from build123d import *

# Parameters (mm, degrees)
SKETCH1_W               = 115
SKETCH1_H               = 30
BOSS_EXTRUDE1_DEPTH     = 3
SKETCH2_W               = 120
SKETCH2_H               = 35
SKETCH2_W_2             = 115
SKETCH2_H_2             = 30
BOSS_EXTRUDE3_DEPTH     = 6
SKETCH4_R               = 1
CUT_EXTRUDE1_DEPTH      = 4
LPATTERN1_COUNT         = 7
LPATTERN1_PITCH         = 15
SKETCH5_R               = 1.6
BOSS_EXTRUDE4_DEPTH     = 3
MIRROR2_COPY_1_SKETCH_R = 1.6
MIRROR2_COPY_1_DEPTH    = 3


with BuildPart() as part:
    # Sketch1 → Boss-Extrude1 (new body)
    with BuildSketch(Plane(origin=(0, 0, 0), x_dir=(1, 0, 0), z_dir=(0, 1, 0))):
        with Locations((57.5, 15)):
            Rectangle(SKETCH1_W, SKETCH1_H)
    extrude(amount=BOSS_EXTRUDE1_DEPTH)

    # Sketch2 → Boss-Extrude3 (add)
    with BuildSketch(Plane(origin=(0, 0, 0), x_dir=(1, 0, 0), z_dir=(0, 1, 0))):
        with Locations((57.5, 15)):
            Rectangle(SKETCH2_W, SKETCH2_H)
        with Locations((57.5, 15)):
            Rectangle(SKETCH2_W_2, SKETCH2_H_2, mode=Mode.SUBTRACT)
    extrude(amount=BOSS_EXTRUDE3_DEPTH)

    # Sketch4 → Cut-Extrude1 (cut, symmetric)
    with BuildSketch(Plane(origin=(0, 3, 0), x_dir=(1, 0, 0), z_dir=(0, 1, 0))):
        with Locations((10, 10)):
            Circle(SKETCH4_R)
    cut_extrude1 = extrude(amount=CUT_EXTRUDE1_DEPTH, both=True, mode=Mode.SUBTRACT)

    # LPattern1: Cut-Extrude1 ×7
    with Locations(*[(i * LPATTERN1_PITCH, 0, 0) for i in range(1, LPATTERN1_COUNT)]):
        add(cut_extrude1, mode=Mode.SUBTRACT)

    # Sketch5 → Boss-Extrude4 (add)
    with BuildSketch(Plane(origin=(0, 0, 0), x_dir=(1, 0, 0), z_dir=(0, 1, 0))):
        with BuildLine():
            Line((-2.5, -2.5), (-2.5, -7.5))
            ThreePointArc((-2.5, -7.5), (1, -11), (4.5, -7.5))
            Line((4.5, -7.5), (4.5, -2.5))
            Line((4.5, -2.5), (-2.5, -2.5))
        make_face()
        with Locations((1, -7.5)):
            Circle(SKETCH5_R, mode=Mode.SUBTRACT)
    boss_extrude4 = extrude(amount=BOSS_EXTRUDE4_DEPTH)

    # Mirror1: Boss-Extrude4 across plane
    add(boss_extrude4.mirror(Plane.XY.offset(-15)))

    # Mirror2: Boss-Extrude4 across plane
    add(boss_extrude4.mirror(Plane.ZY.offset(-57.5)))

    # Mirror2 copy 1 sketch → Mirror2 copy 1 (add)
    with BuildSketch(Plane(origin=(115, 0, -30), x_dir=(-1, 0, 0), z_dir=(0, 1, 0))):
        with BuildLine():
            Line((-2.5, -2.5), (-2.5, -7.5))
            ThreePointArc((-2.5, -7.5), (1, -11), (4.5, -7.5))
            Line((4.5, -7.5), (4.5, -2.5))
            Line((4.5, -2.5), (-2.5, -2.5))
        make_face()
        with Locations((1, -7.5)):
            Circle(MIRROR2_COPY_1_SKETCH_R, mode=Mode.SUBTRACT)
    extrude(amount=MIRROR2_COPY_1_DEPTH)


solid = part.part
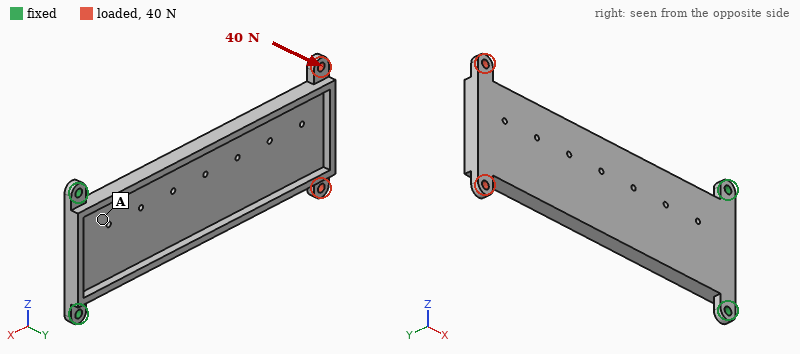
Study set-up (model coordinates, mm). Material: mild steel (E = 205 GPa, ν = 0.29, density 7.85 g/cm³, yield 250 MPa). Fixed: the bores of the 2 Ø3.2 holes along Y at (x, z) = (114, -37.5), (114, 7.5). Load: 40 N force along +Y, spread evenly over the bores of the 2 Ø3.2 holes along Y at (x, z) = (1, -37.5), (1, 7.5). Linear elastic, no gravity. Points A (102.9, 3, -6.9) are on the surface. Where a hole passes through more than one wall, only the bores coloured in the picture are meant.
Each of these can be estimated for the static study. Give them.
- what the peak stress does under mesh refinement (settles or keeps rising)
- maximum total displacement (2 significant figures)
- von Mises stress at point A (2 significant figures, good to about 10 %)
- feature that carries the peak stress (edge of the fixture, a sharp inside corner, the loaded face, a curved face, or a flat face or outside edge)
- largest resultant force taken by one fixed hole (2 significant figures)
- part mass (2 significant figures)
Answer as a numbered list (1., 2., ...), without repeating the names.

1. keeps rising
2. 0.80 mm
3. 26 MPa
4. edge of the fixture
5. 95 N
6. 120 g
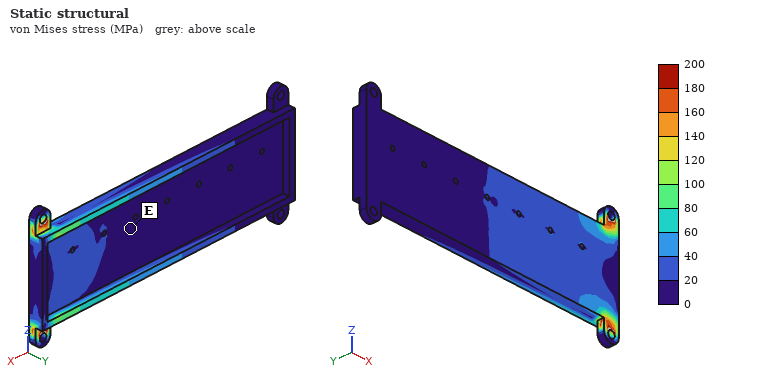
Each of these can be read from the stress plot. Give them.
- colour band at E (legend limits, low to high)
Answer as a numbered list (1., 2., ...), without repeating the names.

1. 0 to 20 MPa
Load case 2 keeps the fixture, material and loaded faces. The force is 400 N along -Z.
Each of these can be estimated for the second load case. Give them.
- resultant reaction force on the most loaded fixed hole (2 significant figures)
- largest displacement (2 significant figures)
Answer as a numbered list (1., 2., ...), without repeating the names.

1. 1.2 kN
2. 0.12 mm
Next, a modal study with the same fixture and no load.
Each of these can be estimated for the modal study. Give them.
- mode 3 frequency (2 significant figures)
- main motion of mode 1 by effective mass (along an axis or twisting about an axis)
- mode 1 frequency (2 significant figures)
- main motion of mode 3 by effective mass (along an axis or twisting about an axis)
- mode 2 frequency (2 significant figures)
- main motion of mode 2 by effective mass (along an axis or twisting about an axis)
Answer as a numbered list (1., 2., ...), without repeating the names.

1. 1300 Hz
2. along Y
3. 190 Hz
4. along Y
5. 1000 Hz
6. twisting about X
